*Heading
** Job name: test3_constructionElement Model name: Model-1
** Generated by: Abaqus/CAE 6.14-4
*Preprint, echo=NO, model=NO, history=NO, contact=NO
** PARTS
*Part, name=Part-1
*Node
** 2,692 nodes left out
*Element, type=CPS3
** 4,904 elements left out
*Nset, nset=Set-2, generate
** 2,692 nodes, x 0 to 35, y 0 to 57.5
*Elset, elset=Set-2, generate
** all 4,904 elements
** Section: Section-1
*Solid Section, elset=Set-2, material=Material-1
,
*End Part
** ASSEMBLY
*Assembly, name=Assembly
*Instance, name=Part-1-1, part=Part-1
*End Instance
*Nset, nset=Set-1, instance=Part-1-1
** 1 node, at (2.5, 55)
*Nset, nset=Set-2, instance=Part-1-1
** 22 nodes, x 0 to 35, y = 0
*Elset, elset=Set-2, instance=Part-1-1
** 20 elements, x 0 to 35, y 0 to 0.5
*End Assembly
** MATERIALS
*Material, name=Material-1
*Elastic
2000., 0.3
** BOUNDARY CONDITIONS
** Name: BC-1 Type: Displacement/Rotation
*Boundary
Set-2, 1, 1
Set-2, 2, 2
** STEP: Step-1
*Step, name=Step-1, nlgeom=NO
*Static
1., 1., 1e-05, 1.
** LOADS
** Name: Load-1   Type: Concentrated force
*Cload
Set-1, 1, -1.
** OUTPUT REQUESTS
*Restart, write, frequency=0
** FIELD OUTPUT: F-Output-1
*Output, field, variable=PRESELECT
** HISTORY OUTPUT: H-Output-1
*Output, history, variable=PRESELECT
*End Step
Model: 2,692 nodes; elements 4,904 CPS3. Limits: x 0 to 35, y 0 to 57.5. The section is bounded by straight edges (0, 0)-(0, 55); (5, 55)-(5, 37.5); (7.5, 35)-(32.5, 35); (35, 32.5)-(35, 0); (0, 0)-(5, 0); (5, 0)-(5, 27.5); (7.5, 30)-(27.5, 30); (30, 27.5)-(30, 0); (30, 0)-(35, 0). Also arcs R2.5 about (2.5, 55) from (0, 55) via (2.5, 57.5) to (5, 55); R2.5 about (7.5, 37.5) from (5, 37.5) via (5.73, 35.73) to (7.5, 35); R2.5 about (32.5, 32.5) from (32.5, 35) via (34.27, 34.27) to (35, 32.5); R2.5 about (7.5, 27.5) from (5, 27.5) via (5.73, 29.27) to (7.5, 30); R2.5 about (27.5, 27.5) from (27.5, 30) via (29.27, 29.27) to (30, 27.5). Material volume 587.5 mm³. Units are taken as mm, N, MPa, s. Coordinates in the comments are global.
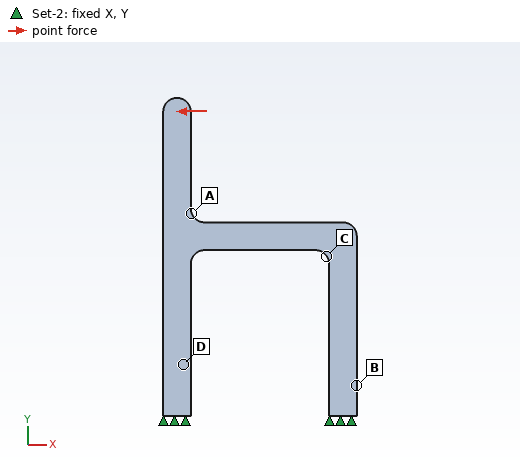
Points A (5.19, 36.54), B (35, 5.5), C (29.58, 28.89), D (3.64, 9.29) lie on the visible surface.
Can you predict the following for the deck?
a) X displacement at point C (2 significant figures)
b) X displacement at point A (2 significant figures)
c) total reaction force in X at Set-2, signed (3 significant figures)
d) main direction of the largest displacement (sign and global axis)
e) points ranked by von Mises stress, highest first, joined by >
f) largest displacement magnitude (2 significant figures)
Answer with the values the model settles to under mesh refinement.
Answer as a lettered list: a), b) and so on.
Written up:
a) -0.11 mm
b) -0.13 mm
c) 1.00 N
d) -X
e) A > C > B > D
f) 0.42 mm
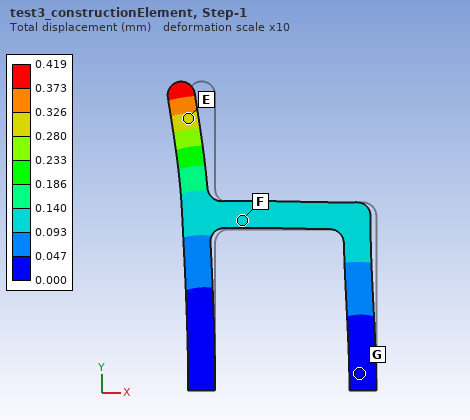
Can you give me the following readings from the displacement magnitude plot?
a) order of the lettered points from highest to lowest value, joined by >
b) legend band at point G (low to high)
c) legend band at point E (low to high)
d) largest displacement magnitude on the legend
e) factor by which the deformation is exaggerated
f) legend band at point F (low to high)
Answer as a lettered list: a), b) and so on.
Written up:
a) E > F > G
b) 0.000 to 0.047 mm
c) 0.280 to 0.326 mm
d) 0.419 mm
e) 10
f) 0.093 to 0.140 mm
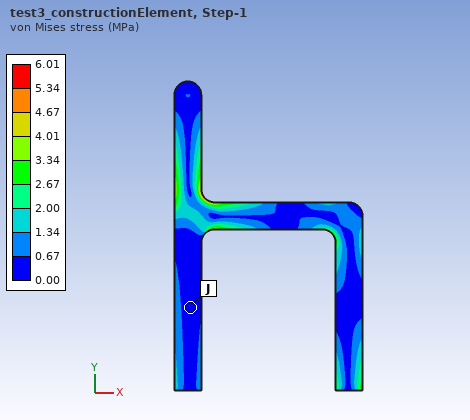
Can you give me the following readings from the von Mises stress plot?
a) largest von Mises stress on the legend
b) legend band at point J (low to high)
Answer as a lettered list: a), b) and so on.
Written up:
a) 6.01 MPa
b) 0.00 to 0.67 MPa
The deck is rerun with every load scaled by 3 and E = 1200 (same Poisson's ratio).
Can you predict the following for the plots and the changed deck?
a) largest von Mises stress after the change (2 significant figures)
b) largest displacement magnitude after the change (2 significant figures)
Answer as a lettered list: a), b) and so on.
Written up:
a) 18 MPa
b) 2.1 mm
